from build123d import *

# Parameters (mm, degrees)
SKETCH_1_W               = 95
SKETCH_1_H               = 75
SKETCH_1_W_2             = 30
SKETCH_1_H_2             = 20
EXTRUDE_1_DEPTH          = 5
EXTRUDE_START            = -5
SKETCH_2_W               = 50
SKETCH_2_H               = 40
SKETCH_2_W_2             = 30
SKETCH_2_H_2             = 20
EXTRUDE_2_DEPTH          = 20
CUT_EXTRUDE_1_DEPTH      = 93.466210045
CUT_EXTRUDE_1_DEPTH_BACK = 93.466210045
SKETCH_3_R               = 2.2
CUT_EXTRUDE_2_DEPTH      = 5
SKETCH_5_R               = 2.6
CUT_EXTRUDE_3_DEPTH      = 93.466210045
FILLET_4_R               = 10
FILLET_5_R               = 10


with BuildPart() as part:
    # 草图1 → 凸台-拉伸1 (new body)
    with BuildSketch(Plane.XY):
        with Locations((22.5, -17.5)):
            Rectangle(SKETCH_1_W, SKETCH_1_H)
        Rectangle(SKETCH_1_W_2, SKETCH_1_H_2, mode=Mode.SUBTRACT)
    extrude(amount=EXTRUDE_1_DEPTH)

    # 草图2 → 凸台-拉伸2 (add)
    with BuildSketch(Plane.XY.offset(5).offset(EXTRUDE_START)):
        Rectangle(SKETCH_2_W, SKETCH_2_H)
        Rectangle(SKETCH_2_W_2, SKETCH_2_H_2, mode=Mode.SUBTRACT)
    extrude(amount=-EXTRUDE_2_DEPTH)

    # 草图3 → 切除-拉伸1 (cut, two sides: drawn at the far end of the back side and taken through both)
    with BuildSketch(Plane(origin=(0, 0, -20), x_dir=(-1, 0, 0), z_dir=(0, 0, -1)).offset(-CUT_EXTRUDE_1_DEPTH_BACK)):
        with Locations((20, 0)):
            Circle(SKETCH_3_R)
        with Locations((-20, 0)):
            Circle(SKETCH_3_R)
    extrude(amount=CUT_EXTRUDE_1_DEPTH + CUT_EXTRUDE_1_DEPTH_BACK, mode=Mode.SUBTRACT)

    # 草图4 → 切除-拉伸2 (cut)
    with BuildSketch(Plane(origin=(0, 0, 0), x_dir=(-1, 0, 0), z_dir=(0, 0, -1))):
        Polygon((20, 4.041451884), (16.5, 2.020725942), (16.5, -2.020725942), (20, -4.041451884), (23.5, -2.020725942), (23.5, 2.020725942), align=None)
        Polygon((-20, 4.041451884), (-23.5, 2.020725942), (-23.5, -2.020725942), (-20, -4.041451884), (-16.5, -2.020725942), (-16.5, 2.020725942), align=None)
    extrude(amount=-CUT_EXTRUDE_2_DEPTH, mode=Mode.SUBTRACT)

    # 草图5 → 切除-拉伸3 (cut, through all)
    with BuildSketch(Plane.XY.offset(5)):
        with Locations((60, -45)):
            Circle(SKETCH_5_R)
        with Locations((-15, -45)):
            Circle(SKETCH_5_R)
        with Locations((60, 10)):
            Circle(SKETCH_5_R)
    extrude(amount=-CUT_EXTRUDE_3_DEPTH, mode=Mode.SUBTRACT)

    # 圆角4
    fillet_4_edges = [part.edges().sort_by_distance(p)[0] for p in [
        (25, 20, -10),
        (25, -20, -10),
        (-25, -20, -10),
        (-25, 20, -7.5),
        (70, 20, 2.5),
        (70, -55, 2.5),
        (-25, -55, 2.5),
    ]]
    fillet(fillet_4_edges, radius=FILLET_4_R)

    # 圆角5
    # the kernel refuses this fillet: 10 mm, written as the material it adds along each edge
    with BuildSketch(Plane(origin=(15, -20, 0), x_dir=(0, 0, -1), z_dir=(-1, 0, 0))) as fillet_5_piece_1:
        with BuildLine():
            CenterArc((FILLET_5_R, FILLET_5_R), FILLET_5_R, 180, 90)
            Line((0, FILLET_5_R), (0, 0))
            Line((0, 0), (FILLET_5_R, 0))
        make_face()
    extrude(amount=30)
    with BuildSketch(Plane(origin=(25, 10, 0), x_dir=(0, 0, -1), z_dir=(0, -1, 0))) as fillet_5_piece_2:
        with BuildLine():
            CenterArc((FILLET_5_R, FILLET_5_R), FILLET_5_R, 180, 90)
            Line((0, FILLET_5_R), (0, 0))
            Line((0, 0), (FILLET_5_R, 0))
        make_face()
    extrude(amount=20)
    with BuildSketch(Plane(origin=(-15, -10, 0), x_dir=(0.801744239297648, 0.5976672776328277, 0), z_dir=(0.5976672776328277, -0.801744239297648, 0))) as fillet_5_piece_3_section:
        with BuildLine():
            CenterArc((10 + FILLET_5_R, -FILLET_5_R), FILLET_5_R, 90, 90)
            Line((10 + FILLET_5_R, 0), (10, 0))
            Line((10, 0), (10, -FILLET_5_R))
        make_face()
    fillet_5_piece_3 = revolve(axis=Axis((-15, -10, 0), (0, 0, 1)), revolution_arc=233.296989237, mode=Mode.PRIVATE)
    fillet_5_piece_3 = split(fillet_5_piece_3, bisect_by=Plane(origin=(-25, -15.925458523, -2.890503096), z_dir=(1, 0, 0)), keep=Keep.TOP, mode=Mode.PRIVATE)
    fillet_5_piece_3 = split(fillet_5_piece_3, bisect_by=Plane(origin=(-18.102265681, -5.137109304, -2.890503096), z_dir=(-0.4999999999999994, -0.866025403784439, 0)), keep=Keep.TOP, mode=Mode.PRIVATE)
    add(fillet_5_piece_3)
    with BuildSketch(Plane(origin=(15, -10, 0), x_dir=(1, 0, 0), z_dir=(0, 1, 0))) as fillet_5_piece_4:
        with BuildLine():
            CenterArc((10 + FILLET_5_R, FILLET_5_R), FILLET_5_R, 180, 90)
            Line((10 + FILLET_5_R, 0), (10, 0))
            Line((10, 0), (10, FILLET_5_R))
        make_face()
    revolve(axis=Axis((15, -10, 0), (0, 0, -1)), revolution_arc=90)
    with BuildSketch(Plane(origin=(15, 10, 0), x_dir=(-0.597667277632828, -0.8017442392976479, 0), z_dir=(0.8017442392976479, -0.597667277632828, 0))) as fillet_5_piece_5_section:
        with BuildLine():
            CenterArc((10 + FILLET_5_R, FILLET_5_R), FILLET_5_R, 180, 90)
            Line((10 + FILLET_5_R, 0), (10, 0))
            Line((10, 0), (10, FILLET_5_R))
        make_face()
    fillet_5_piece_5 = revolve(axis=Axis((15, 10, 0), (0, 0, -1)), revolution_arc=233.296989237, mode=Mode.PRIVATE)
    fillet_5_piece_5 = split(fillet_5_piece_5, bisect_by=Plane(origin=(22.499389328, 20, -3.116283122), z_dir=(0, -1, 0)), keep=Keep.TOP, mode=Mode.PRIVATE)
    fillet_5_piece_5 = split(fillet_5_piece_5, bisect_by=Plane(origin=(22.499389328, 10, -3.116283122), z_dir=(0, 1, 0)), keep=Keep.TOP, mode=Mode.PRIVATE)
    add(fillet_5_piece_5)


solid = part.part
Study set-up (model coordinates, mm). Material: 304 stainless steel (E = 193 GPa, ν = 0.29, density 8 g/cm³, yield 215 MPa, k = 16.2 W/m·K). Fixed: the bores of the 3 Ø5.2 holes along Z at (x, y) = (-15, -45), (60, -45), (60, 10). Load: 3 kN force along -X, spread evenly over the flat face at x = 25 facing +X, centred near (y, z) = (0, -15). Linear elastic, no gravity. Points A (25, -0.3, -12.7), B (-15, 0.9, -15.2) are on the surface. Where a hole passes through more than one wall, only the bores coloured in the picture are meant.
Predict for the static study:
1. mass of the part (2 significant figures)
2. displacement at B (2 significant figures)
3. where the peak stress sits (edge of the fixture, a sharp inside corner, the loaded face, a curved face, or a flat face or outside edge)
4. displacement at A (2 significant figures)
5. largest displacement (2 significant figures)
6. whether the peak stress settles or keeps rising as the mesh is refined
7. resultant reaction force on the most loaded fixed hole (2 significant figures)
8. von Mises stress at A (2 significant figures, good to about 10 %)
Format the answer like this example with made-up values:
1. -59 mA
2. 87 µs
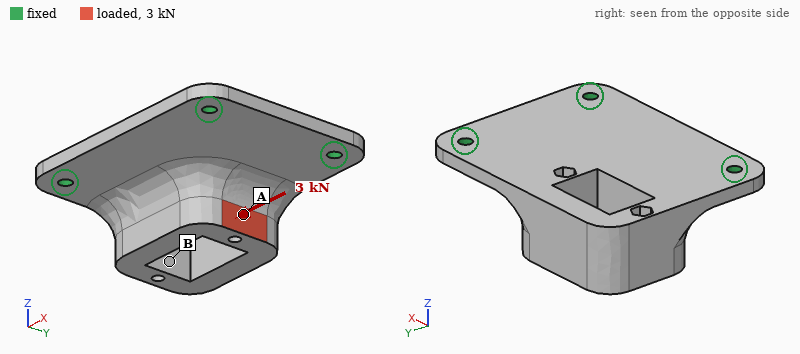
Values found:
1. 470 g
2. 0.079 mm
3. edge of the fixture
4. 0.035 mm
5. 0.11 mm
6. keeps rising
7. 1.4 kN
8. 26 MPa
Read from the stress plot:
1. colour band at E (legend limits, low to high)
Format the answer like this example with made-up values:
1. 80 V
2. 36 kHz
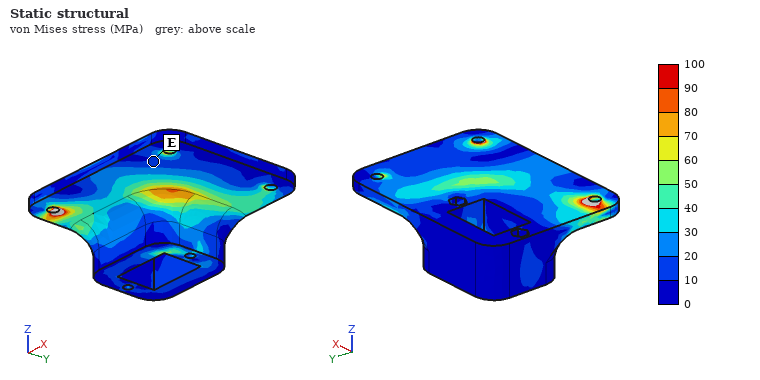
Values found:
1. 10 to 20 MPa
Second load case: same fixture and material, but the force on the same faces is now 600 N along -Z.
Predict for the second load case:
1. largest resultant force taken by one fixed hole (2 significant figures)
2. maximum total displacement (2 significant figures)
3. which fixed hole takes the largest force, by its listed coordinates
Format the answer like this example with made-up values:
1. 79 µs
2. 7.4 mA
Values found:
1. 470 N
2. 36 µm
3. (60, 10)
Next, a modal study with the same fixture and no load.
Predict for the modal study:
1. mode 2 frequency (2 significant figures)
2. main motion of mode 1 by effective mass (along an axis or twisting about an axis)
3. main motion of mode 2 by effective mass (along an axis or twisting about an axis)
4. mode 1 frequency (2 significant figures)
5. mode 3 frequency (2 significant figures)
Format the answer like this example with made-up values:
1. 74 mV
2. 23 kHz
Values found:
1. 3300 Hz
2. along Z
3. along Z
4. 1100 Hz
5. 4400 Hz
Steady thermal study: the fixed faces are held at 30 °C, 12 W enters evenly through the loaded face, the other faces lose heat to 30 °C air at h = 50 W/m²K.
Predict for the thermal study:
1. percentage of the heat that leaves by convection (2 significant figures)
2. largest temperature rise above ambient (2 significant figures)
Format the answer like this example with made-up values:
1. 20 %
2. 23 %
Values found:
1. 83 %
2. 57 K
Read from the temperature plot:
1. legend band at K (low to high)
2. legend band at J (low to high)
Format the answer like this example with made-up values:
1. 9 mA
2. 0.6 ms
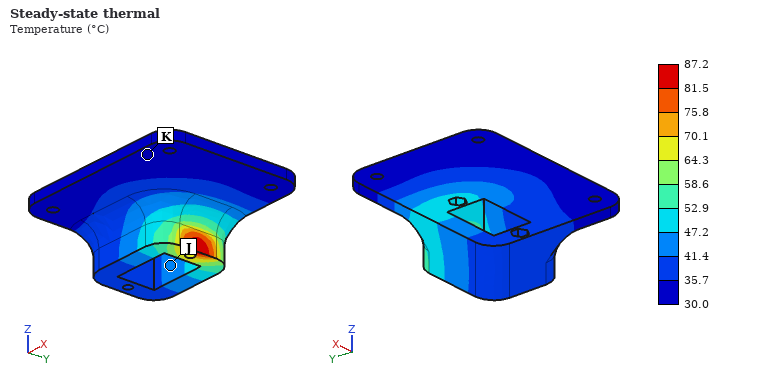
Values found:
1. 30.0 to 35.7 °C
2. 41.4 to 47.2 °C
